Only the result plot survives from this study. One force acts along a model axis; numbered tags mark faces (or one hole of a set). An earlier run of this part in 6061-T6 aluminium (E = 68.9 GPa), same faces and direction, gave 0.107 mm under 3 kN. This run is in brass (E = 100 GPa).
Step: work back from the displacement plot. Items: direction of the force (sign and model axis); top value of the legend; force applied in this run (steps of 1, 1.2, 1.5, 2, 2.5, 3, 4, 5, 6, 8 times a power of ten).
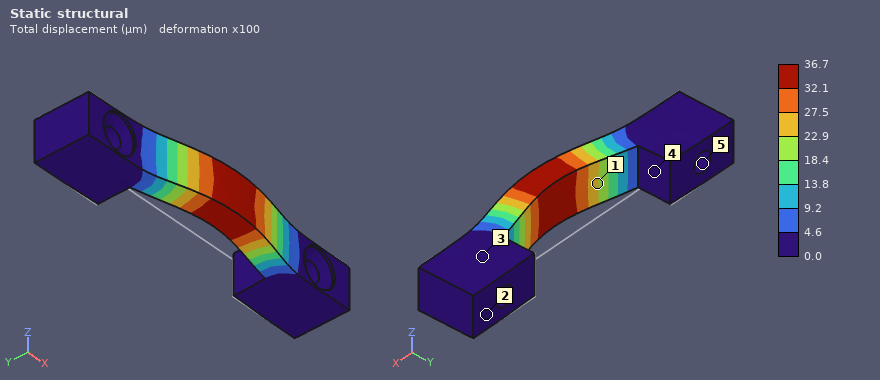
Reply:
-Y
36.7 µm
1.5 kN
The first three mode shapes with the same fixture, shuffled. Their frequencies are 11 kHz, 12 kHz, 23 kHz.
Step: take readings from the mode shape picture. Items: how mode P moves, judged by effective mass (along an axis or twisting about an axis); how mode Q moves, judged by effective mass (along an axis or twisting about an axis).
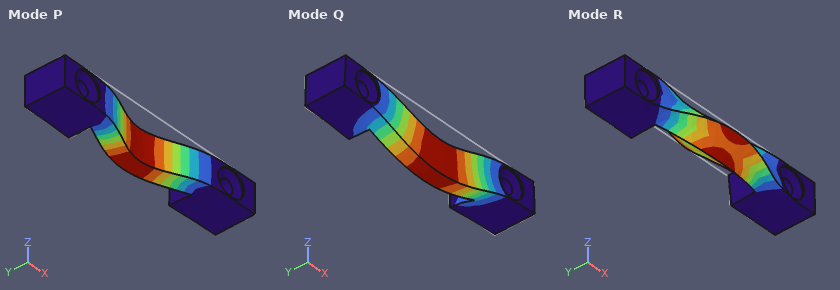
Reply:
along Y
along Z
